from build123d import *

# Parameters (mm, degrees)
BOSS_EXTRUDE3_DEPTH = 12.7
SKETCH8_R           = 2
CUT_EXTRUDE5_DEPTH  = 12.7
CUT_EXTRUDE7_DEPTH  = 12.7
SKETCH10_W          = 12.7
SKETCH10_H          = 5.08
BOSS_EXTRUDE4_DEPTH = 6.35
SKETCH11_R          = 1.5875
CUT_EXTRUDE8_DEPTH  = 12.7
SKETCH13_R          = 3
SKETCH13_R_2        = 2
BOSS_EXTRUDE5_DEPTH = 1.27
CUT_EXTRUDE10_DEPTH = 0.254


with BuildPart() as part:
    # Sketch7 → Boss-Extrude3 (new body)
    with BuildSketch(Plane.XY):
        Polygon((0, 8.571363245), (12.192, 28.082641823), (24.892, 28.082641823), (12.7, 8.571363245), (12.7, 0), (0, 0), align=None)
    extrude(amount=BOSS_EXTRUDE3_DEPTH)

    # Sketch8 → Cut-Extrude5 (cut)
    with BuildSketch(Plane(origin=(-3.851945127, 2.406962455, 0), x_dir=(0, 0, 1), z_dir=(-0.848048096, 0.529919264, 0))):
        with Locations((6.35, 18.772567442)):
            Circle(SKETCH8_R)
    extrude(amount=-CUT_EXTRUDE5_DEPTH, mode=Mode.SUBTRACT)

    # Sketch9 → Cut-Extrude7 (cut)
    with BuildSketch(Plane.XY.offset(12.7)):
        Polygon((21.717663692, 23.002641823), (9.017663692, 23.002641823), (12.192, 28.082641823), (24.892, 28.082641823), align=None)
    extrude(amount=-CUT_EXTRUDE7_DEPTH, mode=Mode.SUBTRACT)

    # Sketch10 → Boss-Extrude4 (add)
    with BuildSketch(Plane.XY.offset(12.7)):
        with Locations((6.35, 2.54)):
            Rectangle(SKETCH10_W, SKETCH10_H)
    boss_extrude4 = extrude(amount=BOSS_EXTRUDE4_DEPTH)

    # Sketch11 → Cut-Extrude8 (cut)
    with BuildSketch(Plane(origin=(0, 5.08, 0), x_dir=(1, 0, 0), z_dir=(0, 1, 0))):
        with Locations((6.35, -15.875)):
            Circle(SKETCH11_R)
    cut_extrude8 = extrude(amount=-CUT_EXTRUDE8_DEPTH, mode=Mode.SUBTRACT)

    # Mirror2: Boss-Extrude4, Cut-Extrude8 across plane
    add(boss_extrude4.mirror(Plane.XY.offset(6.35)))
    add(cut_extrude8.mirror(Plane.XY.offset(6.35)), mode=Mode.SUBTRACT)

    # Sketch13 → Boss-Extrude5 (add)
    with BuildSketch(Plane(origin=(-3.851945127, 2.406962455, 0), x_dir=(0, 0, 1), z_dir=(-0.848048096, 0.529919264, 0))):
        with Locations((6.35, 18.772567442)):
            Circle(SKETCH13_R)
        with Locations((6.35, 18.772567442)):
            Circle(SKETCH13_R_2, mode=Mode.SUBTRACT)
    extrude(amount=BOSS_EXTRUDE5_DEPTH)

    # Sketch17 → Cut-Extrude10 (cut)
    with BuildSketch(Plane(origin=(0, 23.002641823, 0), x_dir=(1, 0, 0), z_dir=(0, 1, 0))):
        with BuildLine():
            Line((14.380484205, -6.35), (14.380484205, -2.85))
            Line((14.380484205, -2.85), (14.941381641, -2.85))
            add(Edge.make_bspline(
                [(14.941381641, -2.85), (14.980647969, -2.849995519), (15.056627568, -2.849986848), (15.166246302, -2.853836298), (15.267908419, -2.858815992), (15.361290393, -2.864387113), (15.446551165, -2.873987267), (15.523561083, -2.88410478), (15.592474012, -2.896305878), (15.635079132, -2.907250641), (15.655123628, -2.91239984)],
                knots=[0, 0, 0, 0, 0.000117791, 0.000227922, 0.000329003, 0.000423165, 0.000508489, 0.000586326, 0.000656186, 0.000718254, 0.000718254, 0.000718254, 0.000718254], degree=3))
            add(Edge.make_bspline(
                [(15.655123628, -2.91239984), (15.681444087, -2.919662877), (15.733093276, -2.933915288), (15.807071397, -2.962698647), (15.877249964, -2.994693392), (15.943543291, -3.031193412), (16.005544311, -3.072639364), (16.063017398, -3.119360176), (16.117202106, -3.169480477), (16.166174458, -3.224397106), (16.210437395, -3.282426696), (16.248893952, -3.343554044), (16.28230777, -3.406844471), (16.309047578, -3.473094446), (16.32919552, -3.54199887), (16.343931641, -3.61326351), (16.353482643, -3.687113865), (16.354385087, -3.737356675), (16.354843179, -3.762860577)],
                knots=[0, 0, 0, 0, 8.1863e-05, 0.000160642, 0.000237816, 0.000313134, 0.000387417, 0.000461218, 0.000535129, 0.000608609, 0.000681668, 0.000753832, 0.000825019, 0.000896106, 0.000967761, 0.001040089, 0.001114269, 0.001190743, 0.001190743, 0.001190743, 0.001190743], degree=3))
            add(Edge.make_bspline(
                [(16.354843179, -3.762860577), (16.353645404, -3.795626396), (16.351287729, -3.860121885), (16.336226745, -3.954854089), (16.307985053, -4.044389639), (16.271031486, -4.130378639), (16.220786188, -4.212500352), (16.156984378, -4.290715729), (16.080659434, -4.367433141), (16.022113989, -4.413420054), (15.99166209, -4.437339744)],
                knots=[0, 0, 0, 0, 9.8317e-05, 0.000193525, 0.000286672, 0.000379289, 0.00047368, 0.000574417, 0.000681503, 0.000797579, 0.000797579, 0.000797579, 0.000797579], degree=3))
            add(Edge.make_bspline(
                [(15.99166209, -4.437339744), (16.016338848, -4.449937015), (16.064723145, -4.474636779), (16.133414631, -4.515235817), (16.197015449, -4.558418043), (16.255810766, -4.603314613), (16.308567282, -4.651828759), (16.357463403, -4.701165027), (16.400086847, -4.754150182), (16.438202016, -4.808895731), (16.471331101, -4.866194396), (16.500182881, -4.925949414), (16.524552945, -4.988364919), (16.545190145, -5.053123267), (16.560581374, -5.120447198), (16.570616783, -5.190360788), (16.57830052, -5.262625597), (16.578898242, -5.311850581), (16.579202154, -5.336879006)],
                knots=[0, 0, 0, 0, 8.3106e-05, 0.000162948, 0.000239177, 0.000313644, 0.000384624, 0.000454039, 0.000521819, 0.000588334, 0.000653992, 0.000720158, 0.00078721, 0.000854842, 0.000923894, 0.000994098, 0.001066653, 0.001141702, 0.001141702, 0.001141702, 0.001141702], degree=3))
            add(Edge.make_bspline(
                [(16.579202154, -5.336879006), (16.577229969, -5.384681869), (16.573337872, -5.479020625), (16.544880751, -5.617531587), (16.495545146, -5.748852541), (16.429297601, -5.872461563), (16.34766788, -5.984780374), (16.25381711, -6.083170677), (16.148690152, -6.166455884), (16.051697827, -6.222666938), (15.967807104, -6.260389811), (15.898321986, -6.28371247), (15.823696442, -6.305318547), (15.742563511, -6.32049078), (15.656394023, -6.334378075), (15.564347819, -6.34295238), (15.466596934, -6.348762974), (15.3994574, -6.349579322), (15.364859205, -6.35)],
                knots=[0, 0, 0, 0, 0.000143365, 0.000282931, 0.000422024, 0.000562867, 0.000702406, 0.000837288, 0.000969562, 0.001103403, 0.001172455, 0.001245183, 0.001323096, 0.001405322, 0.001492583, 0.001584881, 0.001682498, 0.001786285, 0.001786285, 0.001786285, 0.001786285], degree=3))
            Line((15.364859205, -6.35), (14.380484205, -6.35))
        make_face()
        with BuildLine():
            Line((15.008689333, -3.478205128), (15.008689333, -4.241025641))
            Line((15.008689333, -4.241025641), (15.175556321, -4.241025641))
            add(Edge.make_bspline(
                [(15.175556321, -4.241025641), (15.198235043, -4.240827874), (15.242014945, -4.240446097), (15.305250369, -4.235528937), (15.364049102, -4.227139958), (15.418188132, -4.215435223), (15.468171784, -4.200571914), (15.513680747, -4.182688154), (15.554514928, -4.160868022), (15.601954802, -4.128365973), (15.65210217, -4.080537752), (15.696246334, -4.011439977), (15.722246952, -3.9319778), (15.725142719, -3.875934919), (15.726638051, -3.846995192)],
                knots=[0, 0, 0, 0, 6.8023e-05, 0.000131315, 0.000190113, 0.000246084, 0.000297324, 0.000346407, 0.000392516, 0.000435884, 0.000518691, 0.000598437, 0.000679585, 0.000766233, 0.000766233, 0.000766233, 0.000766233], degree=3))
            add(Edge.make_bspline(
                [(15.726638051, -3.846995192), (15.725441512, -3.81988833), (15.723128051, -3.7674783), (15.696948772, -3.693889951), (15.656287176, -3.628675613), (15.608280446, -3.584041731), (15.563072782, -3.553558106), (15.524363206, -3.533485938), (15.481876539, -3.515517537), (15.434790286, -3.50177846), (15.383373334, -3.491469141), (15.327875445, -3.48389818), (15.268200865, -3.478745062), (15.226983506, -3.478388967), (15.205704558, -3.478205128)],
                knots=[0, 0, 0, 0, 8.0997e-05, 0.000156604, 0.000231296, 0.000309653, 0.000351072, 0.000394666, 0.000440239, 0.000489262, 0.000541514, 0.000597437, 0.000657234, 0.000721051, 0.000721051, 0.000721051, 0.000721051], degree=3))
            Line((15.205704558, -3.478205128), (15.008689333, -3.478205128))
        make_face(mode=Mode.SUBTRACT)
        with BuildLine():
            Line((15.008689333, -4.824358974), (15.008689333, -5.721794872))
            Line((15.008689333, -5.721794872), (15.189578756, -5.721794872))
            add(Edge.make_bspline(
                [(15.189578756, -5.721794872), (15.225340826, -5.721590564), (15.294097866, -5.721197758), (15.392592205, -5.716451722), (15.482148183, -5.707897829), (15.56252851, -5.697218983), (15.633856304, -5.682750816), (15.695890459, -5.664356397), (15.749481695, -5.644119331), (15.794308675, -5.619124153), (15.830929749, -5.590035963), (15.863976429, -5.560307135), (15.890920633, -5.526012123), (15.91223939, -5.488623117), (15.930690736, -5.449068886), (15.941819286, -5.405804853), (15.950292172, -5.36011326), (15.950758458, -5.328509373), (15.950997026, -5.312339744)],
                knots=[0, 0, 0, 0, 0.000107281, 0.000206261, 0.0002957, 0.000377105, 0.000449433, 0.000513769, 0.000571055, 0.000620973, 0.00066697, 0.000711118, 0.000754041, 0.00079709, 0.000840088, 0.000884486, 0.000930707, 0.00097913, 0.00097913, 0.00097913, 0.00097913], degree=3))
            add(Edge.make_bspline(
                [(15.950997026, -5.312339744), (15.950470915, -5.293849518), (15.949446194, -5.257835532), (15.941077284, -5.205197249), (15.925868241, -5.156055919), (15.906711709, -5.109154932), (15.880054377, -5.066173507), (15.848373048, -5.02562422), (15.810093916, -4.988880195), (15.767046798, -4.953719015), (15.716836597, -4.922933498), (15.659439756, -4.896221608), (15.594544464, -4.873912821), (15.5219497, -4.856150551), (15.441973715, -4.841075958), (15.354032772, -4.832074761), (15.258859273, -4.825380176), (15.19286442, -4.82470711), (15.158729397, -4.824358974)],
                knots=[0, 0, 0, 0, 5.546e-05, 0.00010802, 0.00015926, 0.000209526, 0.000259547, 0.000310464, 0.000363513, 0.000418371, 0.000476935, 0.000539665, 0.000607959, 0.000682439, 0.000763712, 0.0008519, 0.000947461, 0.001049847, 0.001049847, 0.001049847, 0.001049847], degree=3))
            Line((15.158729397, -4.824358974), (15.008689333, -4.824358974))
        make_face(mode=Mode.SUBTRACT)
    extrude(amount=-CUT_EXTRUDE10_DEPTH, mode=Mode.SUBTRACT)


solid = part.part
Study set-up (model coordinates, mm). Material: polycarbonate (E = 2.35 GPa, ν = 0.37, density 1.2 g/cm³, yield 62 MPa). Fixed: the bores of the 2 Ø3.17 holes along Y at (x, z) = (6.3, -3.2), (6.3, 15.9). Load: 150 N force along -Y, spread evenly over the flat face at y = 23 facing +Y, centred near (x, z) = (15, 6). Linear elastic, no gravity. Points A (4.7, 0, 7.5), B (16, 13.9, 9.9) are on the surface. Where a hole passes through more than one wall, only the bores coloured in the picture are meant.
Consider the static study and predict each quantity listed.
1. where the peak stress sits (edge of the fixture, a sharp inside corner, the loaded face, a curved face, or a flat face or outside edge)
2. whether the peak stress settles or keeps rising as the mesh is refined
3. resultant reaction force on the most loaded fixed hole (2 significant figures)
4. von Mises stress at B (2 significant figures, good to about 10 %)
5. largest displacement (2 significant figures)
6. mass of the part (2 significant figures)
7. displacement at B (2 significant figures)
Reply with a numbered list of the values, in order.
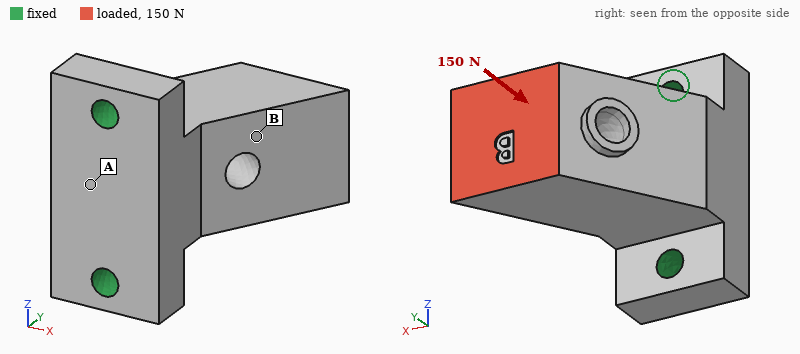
1. edge of the fixture
2. keeps rising
3. 80 N
4. 4.7 MPa
5. 0.31 mm
6. 5.2 g
7. 0.16 mm
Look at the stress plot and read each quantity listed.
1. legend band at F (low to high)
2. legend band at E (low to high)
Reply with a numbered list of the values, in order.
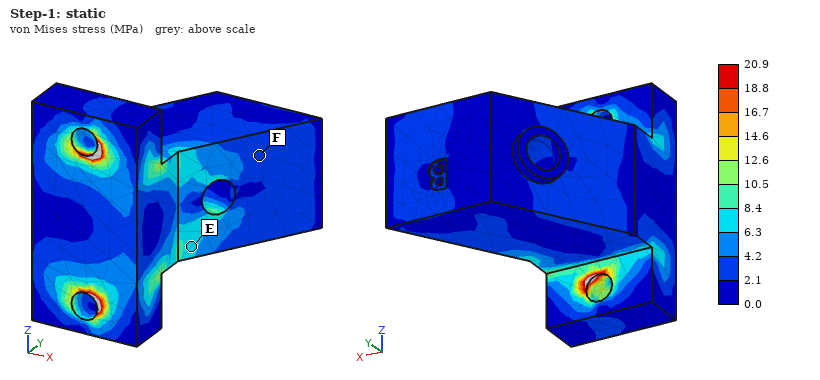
1. 2.1 to 4.2 MPa
2. 6.3 to 8.4 MPa
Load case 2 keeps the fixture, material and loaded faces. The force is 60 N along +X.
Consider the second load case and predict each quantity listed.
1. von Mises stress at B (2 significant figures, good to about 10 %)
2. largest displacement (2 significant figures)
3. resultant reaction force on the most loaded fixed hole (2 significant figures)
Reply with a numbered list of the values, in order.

1. 1.8 MPa
2. 0.25 mm
3. 30 N
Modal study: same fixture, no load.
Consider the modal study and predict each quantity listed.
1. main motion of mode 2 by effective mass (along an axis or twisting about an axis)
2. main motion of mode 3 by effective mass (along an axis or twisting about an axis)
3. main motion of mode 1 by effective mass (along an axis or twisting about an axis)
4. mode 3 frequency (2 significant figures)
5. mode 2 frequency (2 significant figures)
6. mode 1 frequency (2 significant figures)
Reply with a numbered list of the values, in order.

1. along Z
2. along Y
3. along X
4. 8000 Hz
5. 4100 Hz
6. 2300 Hz
